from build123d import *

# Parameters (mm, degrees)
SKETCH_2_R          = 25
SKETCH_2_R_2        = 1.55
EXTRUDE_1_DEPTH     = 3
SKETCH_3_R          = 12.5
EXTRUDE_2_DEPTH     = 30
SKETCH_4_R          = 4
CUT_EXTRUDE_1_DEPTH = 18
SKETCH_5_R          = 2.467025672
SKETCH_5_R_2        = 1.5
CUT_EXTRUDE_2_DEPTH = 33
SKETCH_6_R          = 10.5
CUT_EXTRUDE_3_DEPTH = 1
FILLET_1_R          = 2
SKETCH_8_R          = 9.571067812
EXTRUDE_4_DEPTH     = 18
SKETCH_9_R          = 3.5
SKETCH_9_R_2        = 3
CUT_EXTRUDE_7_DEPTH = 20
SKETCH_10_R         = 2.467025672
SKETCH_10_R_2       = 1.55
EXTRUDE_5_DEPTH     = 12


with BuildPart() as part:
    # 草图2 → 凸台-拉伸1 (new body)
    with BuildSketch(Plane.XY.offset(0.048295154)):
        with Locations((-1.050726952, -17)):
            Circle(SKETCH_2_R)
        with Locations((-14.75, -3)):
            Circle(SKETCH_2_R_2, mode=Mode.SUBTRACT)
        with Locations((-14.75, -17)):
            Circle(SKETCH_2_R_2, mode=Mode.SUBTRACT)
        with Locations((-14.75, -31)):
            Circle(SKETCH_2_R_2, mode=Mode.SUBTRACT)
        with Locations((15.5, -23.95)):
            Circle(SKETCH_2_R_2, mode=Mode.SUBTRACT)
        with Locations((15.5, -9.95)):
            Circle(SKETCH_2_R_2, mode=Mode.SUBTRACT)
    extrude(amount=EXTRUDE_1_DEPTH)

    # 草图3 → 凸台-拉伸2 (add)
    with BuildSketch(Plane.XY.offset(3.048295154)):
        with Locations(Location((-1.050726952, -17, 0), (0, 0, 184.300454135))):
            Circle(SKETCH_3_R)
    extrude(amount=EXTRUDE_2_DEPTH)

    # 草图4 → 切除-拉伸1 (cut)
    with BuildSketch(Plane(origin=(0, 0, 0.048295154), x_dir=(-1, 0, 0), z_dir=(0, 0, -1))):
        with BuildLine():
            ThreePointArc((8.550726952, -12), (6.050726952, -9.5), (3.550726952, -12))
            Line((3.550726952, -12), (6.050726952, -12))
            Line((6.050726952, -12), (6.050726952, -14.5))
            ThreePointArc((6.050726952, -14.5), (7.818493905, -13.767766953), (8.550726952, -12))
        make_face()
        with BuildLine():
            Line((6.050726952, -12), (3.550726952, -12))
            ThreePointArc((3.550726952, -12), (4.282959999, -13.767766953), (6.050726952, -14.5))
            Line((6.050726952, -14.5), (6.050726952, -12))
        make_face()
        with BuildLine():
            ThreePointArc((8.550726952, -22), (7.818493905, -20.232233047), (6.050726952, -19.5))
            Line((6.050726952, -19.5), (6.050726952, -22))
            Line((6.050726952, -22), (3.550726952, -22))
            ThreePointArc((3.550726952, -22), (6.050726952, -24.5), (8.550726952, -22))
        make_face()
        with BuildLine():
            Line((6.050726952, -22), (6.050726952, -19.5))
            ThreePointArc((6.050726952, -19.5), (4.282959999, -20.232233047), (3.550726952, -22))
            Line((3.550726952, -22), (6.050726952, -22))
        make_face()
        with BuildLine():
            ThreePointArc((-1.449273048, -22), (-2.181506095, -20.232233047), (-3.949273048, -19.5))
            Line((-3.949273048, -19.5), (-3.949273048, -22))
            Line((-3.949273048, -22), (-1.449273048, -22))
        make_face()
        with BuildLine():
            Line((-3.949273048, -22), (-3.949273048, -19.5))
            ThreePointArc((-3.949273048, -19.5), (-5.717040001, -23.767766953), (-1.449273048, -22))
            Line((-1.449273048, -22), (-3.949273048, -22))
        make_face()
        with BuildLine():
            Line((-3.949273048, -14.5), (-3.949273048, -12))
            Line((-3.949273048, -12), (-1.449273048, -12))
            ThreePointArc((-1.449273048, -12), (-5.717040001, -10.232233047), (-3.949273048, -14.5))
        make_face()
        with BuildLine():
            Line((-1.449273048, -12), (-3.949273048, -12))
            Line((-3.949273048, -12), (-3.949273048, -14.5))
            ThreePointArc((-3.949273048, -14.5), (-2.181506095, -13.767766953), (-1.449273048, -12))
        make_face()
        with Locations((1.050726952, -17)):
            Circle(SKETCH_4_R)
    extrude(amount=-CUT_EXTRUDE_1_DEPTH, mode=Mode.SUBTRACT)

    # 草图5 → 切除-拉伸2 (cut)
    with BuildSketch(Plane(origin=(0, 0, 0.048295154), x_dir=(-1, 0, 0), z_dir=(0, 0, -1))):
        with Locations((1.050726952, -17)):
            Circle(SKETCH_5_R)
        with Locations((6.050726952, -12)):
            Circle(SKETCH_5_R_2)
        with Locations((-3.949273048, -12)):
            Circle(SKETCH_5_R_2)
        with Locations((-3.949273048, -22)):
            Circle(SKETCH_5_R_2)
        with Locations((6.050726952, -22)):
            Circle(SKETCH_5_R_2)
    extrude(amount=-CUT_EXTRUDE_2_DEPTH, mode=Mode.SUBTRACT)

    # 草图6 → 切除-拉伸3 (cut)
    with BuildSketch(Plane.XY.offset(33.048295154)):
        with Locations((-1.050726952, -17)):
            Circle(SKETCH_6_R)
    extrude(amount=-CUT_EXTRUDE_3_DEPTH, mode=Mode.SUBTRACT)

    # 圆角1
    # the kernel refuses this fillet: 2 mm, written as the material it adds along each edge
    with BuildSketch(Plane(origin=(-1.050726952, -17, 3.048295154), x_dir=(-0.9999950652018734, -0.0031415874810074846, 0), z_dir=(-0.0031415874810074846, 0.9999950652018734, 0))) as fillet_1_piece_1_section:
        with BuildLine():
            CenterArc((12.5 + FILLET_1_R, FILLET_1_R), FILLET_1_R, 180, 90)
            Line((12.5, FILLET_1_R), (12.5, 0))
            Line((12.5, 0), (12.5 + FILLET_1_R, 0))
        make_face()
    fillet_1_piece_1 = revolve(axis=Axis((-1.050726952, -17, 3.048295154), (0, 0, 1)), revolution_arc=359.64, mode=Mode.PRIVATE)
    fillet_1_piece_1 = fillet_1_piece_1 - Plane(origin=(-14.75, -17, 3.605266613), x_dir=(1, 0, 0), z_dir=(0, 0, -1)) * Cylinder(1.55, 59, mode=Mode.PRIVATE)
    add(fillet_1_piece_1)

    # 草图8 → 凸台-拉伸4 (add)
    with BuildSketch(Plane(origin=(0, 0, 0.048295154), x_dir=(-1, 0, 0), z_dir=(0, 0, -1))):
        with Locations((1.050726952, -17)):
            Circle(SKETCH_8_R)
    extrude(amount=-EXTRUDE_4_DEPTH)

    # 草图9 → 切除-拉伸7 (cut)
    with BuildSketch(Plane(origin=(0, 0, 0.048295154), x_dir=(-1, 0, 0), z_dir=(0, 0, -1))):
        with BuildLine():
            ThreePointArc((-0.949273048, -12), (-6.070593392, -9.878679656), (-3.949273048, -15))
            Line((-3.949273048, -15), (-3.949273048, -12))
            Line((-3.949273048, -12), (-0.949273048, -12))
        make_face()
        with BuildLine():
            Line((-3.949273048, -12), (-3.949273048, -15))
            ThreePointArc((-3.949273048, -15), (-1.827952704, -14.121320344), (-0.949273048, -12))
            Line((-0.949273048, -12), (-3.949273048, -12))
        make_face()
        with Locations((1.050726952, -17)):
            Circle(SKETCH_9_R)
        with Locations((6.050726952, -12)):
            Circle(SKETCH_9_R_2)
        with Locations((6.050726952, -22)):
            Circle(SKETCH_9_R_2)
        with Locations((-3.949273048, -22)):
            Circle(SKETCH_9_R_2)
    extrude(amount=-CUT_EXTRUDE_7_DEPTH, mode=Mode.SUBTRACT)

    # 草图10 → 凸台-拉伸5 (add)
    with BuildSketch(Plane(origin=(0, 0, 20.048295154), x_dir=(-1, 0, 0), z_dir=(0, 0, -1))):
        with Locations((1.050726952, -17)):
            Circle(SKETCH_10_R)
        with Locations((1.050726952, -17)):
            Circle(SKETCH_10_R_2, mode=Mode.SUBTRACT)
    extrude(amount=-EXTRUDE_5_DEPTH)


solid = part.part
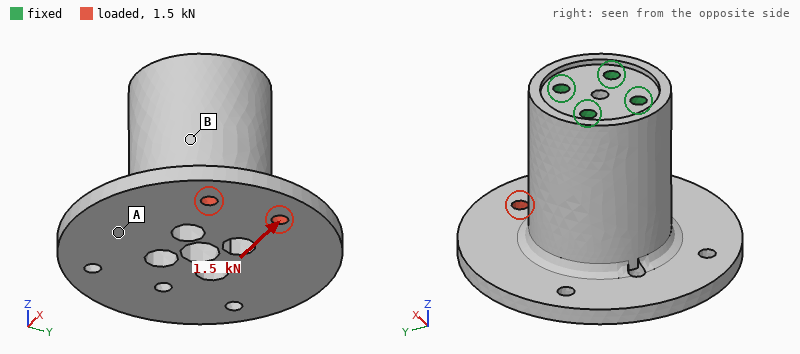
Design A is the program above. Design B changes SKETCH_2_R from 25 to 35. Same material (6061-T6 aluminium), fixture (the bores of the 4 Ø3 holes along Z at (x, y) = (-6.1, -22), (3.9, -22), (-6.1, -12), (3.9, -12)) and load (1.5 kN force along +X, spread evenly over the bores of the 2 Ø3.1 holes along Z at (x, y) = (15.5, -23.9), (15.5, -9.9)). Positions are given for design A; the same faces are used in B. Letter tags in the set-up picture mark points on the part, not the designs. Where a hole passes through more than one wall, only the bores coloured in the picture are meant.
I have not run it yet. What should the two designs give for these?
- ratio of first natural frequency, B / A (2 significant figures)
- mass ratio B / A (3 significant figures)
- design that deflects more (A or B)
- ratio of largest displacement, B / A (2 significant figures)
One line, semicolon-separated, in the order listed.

0.40; 1.34; B; 1.2
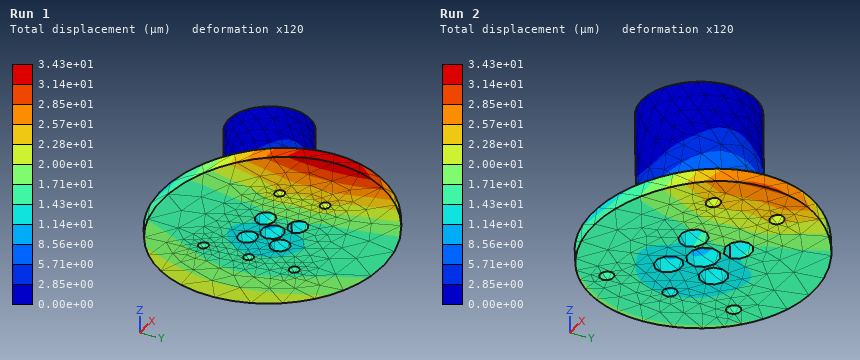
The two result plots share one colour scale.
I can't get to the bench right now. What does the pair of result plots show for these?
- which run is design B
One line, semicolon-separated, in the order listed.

Run 1
